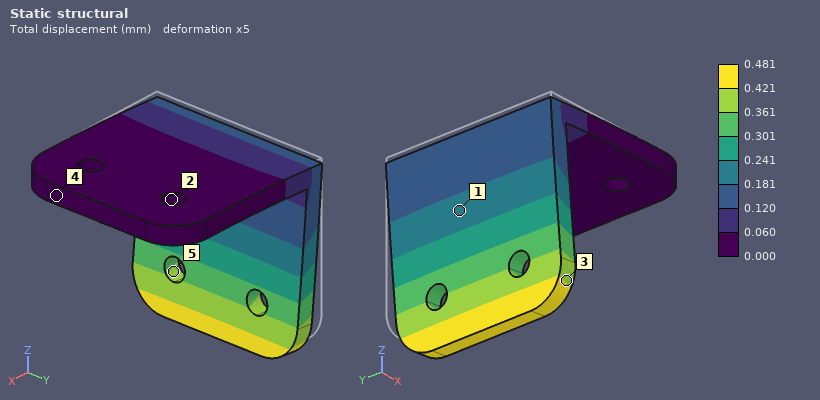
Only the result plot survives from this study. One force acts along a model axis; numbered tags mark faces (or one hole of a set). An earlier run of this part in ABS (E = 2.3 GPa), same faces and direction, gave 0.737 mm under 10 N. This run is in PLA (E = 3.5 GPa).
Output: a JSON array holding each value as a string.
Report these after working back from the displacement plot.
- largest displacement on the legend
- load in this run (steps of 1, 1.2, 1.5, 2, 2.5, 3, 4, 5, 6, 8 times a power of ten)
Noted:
["0.481 mm", "10 N"]
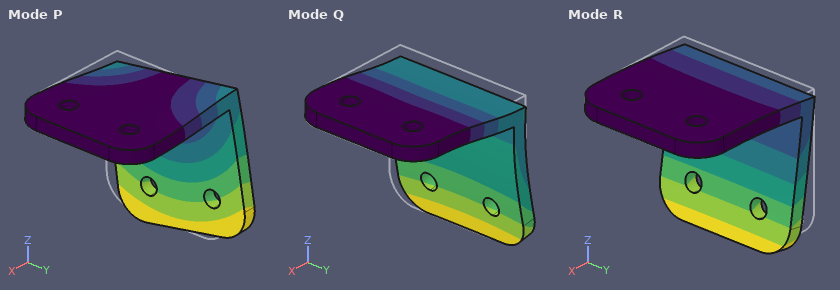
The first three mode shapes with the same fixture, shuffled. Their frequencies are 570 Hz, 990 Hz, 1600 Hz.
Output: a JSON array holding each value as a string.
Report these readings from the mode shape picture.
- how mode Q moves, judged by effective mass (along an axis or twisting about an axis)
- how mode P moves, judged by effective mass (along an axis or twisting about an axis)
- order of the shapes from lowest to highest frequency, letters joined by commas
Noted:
["along Z", "along Y", "R, P, Q"]
